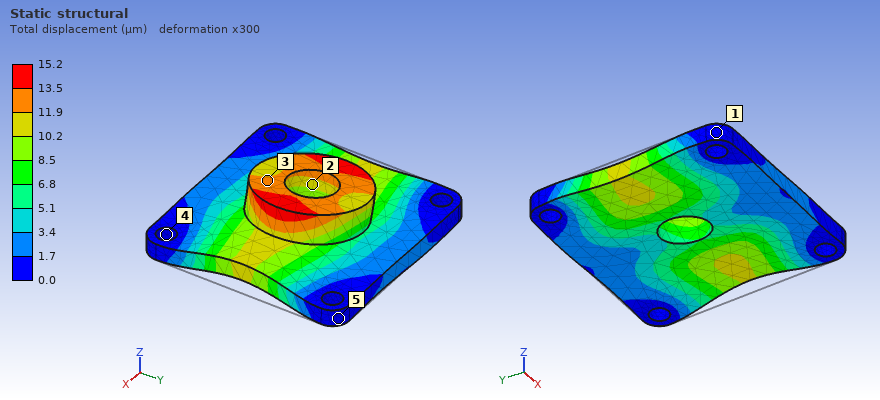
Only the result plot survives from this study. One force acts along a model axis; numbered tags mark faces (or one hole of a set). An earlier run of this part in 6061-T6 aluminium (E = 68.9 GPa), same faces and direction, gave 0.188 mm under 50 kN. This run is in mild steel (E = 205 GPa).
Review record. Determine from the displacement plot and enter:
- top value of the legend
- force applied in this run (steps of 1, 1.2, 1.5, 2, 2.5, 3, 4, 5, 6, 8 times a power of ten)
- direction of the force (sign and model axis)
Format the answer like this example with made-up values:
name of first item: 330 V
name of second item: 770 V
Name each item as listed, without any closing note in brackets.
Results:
top value of the legend: 15.2 µm
force applied in this run: 12 kN
direction of the force: -X
